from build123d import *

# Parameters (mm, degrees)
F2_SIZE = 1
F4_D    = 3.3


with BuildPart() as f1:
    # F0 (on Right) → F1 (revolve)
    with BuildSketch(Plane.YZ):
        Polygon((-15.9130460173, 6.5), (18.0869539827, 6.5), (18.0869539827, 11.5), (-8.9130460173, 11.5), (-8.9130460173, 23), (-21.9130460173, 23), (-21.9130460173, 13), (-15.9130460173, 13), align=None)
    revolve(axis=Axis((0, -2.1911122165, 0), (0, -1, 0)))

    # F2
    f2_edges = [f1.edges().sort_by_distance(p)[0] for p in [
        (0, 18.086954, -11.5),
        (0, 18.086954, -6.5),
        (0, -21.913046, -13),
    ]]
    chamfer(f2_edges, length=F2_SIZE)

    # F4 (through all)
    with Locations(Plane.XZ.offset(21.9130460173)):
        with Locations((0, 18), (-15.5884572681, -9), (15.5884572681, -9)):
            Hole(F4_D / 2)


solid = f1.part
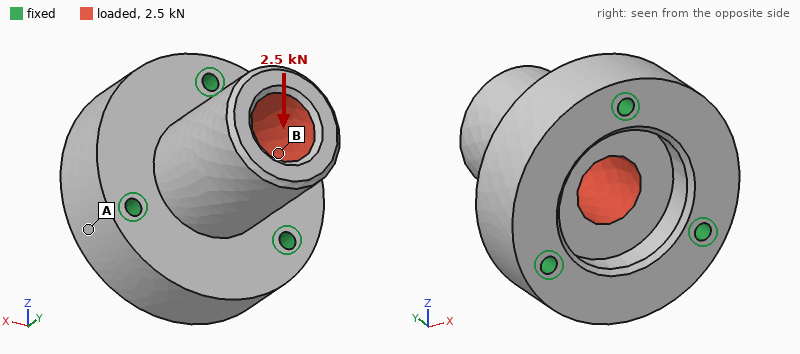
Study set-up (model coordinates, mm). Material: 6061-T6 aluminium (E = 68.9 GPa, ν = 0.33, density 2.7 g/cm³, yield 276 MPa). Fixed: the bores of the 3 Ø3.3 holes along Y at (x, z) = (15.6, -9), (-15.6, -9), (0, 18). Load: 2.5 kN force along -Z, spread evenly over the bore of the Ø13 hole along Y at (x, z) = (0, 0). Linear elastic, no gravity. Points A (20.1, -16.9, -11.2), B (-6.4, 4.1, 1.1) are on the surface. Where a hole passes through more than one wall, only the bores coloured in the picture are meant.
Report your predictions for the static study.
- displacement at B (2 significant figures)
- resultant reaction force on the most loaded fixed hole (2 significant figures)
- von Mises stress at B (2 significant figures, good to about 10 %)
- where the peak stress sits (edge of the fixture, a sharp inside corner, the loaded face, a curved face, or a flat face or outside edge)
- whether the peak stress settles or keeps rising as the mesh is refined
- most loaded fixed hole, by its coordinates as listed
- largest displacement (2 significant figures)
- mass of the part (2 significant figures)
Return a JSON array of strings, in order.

["12 µm", "1.5 kN", "16 MPa", "edge of the fixture", "keeps rising", "(0, 18)", "23 µm", "67 g"]
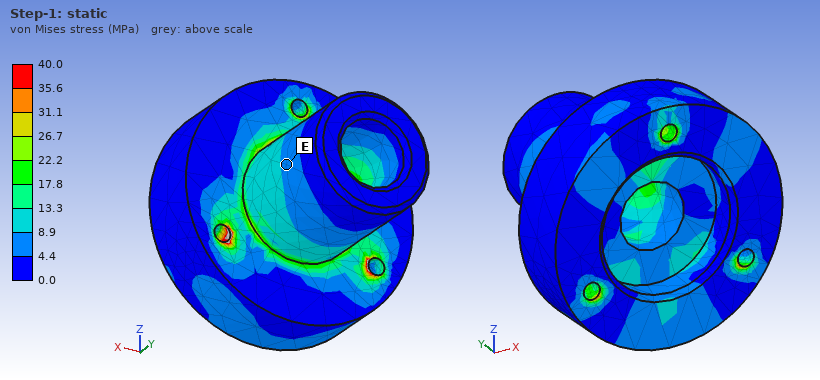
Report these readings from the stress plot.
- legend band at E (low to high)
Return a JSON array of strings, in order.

["4.4 to 8.9 MPa"]
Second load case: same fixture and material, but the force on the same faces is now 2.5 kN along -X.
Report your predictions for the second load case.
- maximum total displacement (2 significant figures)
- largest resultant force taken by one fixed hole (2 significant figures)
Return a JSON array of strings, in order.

["23 µm", "1.4 kN"]
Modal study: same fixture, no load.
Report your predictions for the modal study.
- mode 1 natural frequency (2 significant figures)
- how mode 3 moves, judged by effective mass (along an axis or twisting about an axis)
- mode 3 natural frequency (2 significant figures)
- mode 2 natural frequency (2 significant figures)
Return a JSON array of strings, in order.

["12 kHz", "along Y", "23 kHz", "12 kHz"]
